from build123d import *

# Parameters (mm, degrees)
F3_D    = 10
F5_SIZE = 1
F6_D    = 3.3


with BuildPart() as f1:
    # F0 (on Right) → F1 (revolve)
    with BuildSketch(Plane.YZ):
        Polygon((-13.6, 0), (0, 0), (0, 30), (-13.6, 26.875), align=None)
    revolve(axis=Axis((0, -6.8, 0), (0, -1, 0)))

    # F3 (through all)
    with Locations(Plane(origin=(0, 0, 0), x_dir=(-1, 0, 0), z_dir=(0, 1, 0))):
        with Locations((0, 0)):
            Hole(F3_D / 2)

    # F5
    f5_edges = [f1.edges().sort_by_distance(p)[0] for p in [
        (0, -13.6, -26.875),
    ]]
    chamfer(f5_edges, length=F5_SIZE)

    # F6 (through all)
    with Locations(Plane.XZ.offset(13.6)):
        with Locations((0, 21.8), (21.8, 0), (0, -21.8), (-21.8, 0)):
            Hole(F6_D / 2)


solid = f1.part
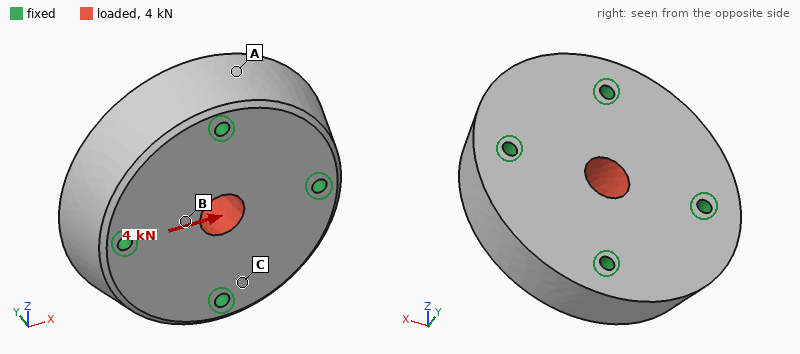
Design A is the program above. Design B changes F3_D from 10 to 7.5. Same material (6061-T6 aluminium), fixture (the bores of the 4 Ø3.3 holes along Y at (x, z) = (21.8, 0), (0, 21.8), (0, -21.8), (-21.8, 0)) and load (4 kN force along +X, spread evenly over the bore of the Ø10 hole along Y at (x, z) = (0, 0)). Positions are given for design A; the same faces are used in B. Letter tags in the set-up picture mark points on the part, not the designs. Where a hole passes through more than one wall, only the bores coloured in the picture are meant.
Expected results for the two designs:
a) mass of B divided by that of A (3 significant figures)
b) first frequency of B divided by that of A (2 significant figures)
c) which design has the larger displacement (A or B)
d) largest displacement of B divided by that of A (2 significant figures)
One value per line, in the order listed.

1.01
1.0
B
1.1
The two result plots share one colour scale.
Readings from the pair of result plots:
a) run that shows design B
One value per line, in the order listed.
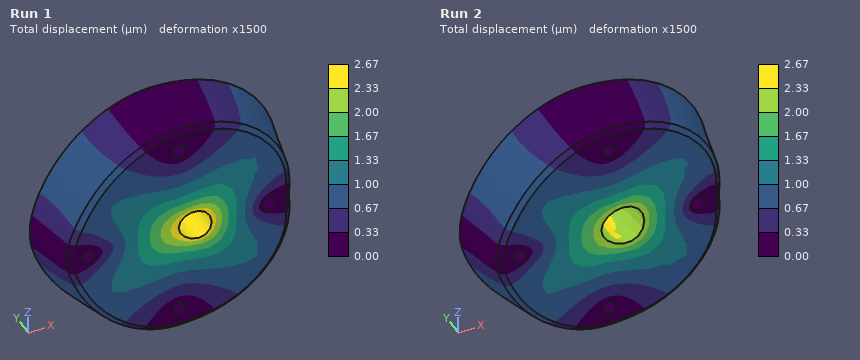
Run 1
